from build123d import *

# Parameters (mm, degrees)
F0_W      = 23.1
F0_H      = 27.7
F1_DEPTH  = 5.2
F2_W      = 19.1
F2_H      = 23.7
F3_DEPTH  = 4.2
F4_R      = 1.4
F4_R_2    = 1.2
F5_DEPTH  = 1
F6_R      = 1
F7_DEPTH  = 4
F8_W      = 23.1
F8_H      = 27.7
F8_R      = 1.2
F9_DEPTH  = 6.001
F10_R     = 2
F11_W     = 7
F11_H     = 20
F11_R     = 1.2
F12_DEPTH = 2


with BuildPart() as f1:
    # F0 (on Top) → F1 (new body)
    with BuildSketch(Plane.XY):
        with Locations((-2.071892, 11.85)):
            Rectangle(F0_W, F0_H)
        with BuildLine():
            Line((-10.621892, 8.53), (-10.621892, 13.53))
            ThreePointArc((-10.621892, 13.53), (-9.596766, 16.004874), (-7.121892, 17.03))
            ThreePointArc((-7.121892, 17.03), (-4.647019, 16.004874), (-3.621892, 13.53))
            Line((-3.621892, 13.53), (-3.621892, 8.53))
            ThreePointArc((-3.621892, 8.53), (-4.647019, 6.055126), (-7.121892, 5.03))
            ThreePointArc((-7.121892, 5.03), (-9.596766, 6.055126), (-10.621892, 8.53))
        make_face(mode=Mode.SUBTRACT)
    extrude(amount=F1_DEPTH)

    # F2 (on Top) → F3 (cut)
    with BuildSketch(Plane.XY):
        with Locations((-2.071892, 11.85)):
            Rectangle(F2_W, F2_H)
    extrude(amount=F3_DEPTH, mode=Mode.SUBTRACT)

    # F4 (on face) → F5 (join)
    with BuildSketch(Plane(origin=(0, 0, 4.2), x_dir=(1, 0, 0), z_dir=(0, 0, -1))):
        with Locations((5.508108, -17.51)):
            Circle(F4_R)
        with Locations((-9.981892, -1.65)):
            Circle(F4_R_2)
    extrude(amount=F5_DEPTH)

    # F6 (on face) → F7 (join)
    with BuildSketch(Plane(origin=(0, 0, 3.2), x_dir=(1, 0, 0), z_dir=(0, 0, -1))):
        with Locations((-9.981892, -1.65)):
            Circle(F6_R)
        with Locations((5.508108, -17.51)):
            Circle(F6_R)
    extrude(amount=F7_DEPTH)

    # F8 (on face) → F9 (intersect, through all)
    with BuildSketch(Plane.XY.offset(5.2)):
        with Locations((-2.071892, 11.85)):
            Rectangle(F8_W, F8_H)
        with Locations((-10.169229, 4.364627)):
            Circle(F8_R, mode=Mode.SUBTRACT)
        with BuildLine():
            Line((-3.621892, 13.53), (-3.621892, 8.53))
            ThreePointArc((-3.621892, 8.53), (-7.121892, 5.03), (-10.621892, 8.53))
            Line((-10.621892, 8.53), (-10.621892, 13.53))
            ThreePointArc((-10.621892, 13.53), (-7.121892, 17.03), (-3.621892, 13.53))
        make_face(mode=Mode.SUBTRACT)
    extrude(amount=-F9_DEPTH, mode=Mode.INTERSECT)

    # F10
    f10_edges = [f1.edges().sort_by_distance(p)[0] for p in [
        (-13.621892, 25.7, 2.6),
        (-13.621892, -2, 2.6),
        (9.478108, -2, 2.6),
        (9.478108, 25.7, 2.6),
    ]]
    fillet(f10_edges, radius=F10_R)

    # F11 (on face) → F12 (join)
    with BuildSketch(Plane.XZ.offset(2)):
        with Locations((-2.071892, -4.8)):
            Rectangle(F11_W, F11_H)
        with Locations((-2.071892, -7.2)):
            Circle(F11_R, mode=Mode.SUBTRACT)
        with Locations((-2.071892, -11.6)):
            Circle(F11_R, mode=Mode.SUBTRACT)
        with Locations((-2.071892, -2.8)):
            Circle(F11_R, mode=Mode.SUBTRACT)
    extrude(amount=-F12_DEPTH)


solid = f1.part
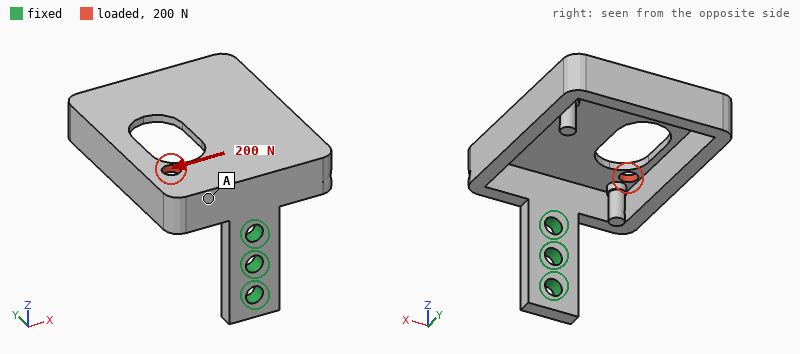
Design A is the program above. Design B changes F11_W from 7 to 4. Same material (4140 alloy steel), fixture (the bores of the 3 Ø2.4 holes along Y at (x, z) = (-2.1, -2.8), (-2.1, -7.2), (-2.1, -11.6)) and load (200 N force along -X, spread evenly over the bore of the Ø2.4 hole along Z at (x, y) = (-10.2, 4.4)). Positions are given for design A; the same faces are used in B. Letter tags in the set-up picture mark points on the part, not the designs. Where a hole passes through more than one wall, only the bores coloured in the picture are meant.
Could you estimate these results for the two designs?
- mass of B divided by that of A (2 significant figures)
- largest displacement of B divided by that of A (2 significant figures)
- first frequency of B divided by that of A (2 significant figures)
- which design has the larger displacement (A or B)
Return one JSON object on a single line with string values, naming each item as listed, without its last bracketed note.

{"mass of B divided by that of A": "0.94", "largest displacement of B divided by that of A": "1.7", "first frequency of B divided by that of A": "0.85", "which design has the larger displacement": "B"}
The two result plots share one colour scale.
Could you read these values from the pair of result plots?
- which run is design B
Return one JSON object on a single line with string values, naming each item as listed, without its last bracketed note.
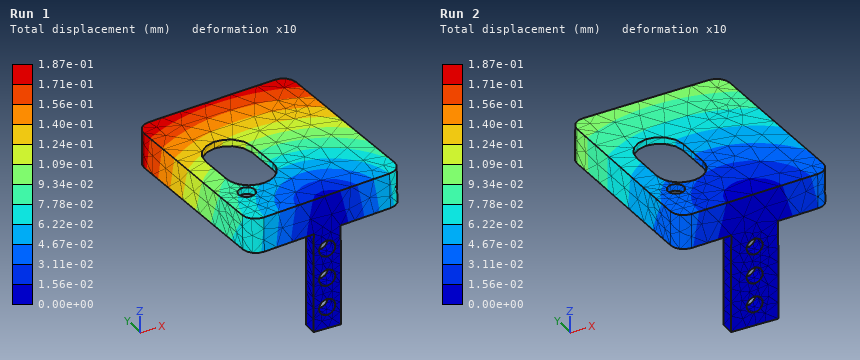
{"which run is design B": "Run 1"}
